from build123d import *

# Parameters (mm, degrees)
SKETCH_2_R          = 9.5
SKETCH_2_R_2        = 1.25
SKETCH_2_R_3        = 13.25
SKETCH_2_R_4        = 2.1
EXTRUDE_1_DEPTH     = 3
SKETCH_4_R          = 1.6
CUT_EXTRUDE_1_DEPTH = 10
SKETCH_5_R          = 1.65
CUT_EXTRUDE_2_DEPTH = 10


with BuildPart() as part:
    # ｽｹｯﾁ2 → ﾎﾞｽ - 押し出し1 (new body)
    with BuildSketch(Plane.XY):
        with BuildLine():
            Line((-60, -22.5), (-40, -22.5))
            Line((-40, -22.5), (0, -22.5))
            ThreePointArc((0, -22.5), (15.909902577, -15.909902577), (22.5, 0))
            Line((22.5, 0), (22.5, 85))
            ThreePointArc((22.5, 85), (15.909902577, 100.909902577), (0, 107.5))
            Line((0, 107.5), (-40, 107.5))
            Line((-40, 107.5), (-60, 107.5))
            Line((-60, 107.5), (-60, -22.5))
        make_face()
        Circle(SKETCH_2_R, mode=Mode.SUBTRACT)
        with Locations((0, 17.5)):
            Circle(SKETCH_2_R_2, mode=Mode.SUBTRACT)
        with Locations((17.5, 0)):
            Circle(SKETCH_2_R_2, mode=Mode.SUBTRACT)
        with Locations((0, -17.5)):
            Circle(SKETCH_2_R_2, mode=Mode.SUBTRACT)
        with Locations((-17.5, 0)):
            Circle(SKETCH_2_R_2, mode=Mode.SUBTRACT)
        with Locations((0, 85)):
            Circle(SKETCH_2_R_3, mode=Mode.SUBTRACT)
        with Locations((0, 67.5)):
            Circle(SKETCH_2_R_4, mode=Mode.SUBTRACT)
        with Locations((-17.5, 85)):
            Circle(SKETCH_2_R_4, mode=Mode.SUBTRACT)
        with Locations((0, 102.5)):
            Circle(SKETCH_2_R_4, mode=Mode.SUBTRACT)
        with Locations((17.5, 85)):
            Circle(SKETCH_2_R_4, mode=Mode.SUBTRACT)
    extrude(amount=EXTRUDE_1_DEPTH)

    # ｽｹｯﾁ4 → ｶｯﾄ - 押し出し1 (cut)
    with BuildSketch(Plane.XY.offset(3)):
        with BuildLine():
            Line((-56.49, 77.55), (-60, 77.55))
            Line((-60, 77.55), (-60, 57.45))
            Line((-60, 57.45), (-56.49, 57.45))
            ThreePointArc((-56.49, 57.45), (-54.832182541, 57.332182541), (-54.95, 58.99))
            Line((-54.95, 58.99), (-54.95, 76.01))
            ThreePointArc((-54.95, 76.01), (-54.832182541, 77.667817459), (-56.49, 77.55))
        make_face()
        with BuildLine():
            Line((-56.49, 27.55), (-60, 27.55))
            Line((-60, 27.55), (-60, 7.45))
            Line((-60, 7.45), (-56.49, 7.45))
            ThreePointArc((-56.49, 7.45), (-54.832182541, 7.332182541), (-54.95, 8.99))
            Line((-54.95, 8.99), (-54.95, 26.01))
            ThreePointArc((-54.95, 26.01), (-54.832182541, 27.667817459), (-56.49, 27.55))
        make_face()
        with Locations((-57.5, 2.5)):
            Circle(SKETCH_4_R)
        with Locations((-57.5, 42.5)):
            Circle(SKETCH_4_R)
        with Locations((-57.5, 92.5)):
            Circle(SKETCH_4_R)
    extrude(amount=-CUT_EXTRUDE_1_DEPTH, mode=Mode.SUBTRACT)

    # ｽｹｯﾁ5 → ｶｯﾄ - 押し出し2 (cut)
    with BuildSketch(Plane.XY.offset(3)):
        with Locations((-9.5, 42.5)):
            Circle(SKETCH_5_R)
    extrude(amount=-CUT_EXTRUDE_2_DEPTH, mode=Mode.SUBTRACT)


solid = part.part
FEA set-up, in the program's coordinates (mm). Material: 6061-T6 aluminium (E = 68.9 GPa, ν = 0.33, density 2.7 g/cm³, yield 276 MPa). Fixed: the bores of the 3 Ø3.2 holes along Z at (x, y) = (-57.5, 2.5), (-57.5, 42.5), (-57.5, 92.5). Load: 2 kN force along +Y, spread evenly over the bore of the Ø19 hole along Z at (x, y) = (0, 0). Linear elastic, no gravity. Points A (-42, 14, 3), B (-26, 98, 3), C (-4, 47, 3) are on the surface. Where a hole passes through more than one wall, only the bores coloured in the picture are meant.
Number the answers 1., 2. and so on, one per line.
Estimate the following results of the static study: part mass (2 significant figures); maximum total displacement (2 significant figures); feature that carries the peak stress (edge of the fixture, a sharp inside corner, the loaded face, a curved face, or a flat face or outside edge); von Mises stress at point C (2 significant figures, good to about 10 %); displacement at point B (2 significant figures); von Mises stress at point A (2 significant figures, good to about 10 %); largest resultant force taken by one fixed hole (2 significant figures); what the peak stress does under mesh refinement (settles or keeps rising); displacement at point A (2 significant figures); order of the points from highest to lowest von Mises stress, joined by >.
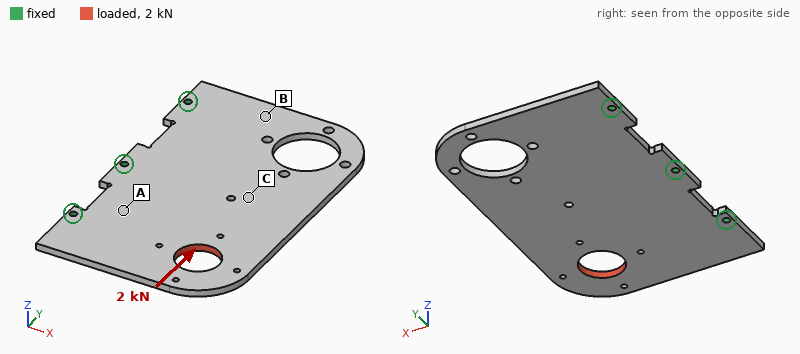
1. 76 g
2. 49 µm
3. edge of the fixture
4. 12 MPa
5. 17 µm
6. 21 MPa
7. 1.4 kN
8. keeps rising
9. 11 µm
10. A > C > B
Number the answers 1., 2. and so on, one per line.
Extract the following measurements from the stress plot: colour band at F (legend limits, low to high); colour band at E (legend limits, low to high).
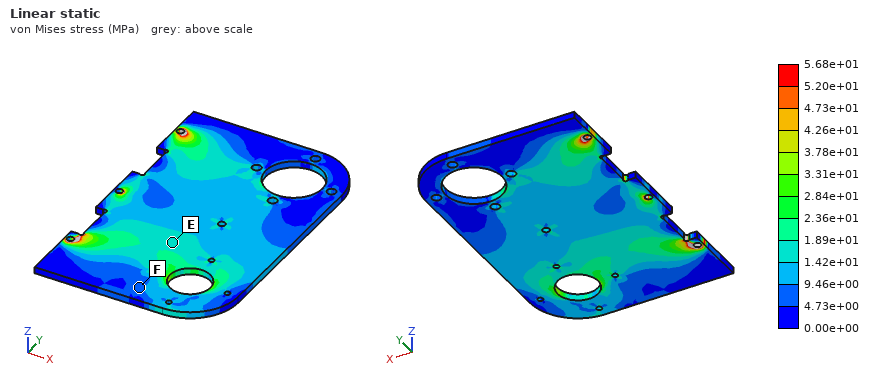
1. 4.73e+00 to 9.46e+00 MPa
2. 1.42e+01 to 1.89e+01 MPa
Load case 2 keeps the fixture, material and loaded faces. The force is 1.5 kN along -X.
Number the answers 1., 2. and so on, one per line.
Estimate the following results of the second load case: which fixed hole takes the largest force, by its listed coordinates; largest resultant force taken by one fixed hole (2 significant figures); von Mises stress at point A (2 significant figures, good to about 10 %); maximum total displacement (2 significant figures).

1. (-57.5, 2.5)
2. 1.3 kN
3. 9.4 MPa
4. 24 µm
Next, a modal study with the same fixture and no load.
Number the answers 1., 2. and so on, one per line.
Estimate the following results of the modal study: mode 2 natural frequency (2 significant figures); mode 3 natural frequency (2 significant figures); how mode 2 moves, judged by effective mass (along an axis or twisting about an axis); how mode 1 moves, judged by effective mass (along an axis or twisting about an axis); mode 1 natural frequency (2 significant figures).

1. 700 Hz
2. 1400 Hz
3. twisting about X
4. along Z
5. 350 Hz
